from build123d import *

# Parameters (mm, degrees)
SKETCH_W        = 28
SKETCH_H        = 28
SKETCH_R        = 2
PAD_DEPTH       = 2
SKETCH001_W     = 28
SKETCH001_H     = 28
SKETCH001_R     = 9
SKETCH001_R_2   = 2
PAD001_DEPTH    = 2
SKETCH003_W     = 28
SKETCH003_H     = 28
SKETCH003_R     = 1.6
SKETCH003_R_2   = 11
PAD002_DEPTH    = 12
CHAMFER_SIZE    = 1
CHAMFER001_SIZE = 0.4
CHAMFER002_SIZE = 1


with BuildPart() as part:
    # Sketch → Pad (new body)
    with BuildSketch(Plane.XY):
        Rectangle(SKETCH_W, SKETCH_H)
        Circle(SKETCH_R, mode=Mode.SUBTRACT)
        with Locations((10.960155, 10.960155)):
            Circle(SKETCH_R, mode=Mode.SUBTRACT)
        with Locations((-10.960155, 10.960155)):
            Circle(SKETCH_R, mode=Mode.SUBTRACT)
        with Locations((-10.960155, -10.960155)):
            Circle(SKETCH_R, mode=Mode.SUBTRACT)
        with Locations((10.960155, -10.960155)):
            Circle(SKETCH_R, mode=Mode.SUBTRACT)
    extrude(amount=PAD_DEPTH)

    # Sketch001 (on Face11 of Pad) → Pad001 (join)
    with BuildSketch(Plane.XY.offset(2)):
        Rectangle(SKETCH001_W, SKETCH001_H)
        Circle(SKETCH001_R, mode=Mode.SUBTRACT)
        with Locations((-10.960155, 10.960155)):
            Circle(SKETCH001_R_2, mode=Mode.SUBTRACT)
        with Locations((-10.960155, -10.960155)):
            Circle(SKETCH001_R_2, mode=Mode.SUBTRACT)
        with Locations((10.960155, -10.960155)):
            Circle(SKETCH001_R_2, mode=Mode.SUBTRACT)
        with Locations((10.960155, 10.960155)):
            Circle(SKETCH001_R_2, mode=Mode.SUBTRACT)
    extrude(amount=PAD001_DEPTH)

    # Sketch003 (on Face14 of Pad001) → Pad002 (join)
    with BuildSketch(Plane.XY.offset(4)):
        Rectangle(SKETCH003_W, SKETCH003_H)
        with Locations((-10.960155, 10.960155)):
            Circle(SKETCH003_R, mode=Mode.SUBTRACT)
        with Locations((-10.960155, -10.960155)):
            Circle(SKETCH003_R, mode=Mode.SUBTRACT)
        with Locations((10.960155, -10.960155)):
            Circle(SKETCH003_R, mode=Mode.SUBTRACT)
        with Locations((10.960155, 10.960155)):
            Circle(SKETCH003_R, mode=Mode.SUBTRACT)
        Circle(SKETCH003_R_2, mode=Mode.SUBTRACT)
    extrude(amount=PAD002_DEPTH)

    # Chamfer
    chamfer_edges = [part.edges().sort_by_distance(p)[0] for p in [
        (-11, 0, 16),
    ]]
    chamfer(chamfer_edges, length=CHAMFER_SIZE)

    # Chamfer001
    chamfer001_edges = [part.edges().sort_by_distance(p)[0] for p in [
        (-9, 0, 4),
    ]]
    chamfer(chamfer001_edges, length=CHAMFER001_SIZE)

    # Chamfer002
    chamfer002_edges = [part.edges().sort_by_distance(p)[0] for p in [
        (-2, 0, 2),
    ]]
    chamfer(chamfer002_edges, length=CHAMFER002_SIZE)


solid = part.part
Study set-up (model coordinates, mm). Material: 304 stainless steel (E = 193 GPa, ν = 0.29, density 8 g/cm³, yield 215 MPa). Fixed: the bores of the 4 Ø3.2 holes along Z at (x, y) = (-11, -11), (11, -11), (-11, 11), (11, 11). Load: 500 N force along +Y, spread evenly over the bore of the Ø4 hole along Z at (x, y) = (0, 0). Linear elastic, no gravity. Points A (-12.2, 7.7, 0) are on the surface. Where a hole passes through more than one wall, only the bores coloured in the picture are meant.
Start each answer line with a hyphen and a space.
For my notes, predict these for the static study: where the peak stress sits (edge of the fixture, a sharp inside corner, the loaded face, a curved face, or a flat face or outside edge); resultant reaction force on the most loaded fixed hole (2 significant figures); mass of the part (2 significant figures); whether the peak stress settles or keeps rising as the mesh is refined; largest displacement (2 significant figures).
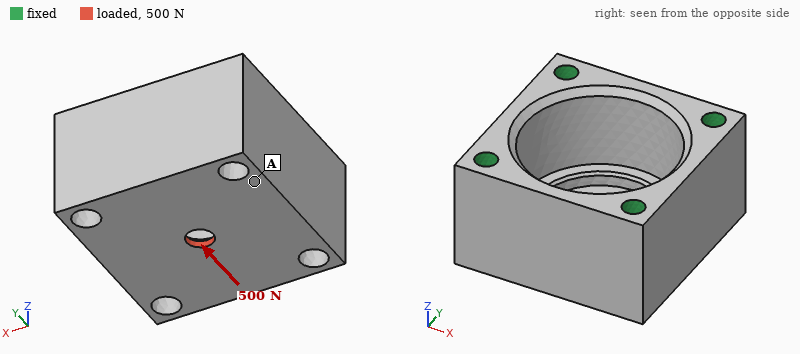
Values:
- a sharp inside corner
- 140 N
- 55 g
- keeps rising
- 1.2 µm
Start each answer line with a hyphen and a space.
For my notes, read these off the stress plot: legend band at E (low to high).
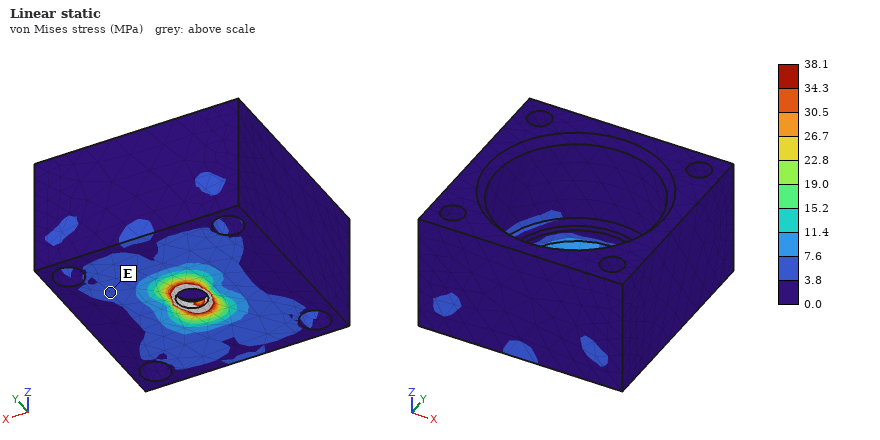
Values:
- 3.8 to 7.6 MPa
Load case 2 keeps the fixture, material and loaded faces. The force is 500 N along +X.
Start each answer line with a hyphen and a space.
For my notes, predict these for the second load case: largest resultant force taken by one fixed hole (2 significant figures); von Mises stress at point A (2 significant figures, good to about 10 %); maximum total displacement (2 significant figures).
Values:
- 140 N
- 3.9 MPa
- 1.2 µm
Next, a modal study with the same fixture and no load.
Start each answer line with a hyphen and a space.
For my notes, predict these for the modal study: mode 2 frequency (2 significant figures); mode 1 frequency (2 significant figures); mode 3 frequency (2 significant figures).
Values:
- 50 kHz
- 40 kHz
- 51 kHz
